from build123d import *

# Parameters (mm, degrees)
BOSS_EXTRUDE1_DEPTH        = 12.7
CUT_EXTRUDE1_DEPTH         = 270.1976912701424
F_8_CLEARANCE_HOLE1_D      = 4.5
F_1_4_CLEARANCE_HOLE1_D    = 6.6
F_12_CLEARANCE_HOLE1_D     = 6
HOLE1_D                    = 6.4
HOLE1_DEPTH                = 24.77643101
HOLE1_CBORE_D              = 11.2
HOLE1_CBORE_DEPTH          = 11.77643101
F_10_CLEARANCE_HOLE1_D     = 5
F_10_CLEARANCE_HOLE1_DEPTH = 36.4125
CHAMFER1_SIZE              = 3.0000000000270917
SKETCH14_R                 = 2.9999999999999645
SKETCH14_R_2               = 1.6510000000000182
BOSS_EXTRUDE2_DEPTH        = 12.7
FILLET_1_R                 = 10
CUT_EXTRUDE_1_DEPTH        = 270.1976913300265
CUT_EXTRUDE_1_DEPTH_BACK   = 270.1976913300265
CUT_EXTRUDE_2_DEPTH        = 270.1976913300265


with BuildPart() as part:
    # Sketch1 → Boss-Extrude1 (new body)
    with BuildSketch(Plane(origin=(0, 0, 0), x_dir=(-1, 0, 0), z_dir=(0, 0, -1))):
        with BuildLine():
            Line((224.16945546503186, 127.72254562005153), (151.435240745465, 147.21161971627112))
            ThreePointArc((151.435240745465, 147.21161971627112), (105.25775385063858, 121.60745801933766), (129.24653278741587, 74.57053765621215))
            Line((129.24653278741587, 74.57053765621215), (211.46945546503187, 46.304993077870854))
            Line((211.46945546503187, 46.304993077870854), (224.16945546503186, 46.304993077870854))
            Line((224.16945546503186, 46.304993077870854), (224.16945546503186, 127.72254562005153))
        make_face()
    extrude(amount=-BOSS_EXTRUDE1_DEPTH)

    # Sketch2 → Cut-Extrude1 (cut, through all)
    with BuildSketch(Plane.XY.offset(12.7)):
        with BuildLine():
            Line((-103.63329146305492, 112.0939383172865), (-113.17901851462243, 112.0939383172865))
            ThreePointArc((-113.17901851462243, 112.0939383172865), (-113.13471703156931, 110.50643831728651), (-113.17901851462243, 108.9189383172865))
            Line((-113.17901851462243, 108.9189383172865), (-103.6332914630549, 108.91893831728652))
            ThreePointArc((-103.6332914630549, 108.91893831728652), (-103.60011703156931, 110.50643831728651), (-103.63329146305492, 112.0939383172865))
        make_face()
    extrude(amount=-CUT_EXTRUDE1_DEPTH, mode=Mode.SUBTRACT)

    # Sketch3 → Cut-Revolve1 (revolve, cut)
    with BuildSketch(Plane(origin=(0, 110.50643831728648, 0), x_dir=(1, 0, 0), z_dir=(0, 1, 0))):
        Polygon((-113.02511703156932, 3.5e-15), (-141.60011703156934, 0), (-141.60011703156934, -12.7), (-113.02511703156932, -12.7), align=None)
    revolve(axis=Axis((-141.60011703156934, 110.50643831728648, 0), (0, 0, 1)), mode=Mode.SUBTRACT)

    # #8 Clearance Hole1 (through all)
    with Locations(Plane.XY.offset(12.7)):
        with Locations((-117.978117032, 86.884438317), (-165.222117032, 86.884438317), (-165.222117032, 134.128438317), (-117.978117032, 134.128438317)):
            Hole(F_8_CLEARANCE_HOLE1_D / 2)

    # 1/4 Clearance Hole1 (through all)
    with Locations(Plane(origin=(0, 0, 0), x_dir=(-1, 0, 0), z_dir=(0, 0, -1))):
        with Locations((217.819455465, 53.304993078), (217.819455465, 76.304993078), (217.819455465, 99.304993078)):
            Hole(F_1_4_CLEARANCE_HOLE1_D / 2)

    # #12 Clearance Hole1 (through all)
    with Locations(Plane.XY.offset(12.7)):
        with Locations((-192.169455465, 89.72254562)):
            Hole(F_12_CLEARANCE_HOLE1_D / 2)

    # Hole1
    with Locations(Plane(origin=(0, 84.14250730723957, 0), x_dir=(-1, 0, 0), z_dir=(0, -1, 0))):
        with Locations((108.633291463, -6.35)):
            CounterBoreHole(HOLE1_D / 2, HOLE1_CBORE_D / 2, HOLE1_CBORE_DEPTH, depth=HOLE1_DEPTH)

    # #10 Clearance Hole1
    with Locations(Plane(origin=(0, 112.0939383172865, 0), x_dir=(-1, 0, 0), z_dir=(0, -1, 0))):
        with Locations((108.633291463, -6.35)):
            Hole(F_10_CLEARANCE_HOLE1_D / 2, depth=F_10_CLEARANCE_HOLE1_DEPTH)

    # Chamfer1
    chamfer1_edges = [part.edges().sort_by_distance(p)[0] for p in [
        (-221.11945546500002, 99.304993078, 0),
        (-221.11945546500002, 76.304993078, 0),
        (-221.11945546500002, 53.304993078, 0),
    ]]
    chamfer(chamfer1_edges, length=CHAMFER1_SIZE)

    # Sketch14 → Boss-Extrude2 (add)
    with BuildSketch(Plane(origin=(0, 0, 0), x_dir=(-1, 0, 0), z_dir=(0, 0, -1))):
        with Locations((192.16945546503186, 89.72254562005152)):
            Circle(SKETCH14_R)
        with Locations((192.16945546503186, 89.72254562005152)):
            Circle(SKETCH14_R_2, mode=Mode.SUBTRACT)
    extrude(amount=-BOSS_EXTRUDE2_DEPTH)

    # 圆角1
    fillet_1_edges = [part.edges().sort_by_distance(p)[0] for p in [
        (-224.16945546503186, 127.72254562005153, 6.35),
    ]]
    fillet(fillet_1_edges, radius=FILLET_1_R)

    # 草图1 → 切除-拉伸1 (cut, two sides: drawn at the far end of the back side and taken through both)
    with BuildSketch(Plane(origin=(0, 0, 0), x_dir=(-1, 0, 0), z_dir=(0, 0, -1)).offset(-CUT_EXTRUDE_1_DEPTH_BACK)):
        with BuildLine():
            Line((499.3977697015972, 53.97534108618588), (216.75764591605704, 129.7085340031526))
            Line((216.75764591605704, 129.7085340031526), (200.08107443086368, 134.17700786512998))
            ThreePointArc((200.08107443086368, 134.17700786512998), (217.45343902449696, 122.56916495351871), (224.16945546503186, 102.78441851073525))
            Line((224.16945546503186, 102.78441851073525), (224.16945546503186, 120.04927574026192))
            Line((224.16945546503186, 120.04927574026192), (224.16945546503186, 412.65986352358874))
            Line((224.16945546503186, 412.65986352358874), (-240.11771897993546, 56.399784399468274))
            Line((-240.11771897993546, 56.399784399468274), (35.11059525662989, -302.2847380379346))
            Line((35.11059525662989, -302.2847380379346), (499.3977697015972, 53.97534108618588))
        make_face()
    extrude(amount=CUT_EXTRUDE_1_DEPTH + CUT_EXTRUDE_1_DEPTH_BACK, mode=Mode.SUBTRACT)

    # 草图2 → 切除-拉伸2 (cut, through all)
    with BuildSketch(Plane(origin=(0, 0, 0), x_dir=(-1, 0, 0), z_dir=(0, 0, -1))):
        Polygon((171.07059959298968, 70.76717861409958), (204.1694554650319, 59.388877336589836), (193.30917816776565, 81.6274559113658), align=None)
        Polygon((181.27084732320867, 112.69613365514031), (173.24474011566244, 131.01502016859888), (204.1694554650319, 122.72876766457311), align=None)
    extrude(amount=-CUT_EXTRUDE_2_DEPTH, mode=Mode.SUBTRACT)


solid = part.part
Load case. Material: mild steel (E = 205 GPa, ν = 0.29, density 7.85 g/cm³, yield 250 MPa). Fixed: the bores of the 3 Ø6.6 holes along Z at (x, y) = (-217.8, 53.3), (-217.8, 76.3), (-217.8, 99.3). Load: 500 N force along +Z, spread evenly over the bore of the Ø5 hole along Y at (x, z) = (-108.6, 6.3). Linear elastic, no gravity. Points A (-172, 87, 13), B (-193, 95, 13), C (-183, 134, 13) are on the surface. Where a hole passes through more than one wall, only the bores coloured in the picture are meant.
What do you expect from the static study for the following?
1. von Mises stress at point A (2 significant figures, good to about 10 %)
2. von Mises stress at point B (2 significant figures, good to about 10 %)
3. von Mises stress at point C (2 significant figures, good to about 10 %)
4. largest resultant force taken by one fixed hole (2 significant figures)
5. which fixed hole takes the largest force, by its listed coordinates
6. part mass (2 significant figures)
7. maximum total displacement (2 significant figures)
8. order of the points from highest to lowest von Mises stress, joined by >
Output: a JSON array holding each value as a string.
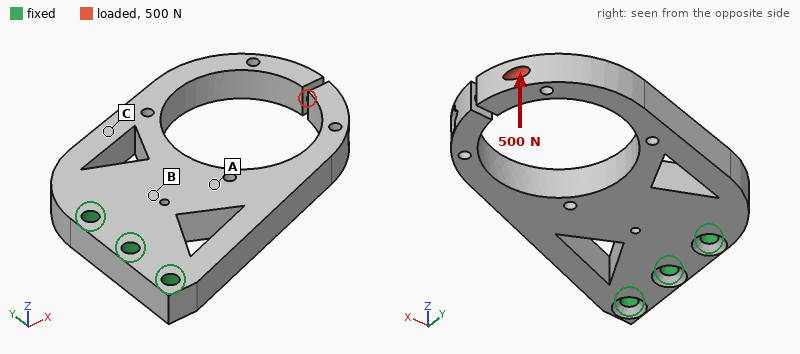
["13 MPa", "33 MPa", "66 MPa", "610 N", "(-217.8, 99.3)", "550 g", "0.47 mm", "C > B > A"]
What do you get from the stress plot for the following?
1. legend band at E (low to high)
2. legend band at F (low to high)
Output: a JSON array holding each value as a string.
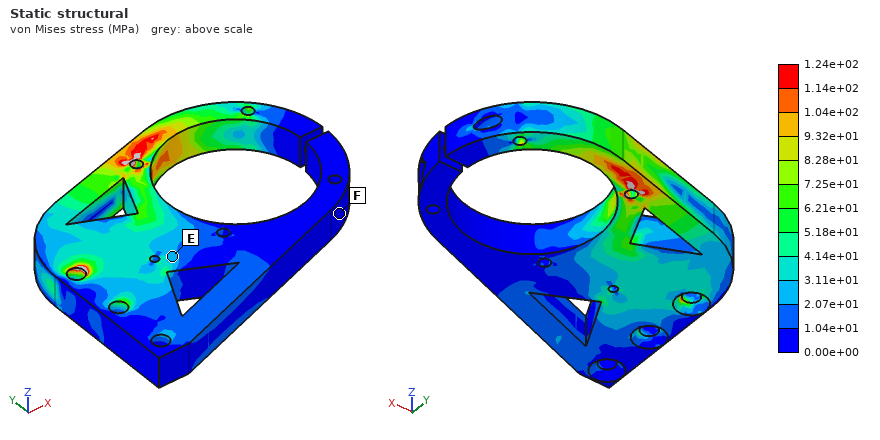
["2.07e+01 to 3.11e+01 MPa", "0.00e+00 to 1.04e+01 MPa"]
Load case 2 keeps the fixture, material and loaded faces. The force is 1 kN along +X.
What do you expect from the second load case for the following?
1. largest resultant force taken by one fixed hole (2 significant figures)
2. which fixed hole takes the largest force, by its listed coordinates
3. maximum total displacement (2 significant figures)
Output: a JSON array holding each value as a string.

["1.4 kN", "(-217.8, 99.3)", "0.28 mm"]
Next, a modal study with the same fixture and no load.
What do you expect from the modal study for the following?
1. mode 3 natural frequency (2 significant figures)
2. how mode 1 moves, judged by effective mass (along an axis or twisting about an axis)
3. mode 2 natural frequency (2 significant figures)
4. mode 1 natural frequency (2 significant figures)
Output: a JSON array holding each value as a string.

["1500 Hz", "along Z", "1500 Hz", "930 Hz"]
